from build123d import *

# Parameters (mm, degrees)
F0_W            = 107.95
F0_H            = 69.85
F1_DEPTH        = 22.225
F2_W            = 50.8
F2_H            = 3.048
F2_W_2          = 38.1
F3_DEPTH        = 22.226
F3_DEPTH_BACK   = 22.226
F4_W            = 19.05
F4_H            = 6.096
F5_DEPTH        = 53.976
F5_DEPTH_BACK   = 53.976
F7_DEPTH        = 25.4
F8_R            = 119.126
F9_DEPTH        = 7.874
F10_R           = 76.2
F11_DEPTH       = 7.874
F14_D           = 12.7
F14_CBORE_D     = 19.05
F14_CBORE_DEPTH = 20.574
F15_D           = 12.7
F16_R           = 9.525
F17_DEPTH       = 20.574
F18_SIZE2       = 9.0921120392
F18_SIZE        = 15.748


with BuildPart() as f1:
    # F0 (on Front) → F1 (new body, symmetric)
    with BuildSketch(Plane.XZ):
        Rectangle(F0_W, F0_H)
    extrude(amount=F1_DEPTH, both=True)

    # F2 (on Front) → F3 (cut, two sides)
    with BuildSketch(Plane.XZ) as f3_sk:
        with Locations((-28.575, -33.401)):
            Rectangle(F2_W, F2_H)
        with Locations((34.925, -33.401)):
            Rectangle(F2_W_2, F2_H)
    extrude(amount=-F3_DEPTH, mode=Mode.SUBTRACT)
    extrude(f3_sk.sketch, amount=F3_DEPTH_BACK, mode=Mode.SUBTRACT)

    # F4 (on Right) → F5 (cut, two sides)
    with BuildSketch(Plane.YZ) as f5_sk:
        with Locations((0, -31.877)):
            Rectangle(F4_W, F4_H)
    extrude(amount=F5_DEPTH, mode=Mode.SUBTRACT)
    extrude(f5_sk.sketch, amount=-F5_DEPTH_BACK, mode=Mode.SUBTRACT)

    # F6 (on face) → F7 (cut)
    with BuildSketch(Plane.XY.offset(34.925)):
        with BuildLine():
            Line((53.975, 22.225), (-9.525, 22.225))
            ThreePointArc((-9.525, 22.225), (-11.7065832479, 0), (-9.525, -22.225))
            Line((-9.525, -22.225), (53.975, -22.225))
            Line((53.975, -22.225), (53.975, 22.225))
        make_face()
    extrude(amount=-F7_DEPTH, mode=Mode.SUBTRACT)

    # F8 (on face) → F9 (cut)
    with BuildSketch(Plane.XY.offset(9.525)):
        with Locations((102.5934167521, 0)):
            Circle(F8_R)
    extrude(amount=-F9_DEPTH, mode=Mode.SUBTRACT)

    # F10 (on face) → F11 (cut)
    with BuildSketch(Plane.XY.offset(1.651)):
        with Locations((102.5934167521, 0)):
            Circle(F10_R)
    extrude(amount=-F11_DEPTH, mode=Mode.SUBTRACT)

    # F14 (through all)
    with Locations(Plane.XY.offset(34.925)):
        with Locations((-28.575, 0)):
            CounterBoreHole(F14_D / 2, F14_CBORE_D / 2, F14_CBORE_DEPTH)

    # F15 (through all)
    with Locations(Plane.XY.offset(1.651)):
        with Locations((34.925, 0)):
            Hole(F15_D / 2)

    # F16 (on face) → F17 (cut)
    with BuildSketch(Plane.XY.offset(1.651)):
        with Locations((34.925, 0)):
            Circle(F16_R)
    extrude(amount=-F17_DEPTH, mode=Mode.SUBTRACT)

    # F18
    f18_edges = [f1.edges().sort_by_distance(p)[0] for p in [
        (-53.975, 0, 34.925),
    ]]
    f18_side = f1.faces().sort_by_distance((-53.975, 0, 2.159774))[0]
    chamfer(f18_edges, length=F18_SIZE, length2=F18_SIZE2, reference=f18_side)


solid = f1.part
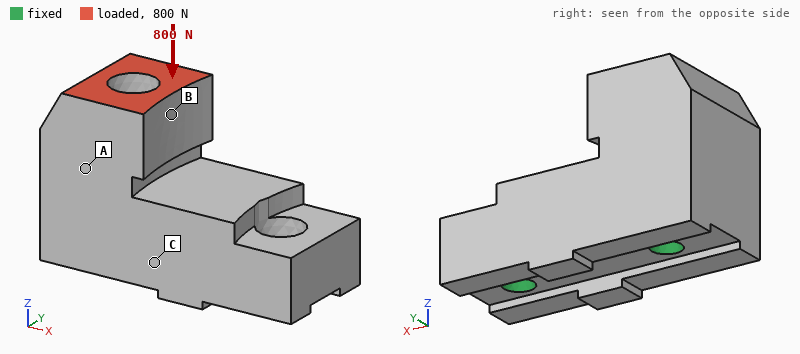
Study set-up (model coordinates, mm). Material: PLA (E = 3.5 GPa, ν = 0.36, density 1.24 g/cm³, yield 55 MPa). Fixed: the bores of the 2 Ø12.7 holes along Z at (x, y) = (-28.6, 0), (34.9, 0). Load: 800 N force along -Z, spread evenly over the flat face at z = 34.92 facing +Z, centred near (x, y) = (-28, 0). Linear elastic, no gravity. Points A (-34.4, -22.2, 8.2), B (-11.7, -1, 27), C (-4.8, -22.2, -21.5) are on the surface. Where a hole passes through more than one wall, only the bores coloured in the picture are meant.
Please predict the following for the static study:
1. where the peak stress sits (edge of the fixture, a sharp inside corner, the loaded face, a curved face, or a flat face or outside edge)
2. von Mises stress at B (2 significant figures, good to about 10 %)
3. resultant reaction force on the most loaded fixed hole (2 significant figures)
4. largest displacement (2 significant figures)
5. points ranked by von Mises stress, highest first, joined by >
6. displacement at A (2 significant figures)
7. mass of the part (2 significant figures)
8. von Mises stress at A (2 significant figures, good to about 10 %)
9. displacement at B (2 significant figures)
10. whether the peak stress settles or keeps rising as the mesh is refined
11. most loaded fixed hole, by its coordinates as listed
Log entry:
edge of the fixture
0.74 MPa
780 N
13 µm
B > A > C
3.7 µm
230 g
0.38 MPa
9.7 µm
keeps rising
(-28.6, 0)
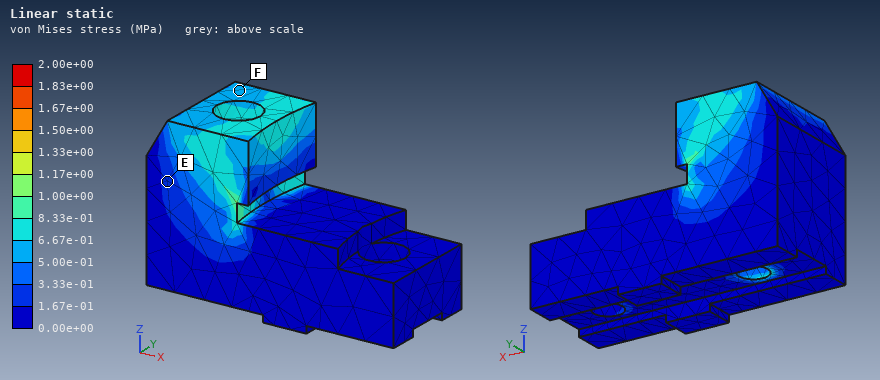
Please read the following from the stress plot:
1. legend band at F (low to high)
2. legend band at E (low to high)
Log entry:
5.00e-01 to 6.67e-01 MPa
1.67e-01 to 3.33e-01 MPa
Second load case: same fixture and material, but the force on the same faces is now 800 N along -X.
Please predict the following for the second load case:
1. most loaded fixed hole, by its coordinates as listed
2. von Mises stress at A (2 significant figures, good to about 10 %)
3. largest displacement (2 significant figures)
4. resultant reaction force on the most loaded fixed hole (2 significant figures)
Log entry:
(-28.6, 0)
0.63 MPa
60 µm
780 N
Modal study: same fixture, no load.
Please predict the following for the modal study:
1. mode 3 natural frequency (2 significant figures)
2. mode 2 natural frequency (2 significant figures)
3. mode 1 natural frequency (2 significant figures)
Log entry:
4500 Hz
4400 Hz
3700 Hz
